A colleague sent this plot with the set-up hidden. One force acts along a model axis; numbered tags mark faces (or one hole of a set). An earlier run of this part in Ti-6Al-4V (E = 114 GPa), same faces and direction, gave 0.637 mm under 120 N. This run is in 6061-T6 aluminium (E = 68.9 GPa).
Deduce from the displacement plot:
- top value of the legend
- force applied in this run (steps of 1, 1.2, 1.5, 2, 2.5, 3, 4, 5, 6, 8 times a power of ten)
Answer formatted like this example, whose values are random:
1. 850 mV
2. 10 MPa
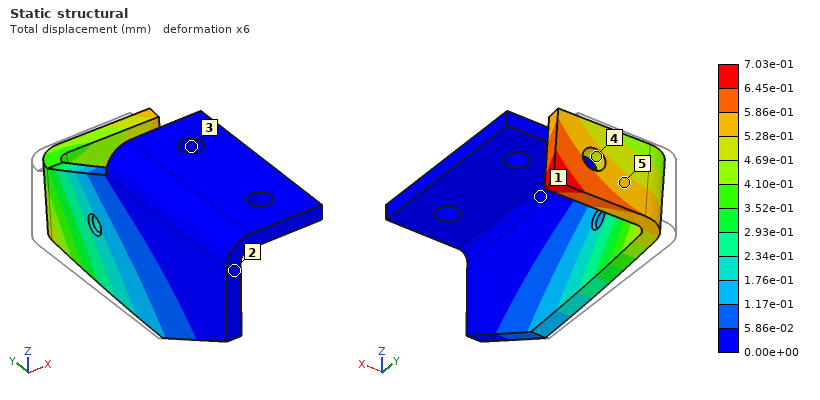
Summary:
1. 7.03e-01 mm
2. 80 N
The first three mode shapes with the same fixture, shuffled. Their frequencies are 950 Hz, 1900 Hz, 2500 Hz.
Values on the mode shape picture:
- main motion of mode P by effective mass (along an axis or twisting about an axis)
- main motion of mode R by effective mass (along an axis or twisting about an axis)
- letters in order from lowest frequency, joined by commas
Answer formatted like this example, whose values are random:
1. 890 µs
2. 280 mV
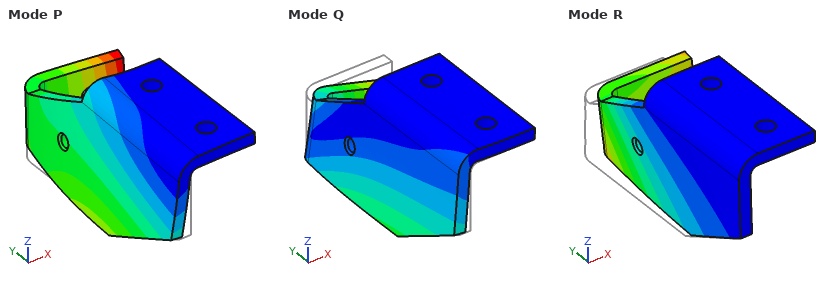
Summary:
1. along Z
2. along X
3. R, Q, P
